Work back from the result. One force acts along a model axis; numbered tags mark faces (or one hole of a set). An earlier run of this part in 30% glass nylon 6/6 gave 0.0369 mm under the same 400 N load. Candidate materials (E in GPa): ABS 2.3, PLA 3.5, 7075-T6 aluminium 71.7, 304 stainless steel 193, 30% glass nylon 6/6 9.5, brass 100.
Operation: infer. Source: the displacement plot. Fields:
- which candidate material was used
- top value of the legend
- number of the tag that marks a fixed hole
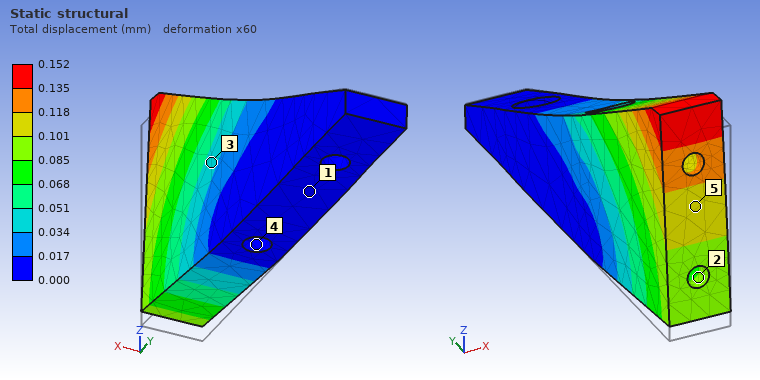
ABS
0.152 mm
4
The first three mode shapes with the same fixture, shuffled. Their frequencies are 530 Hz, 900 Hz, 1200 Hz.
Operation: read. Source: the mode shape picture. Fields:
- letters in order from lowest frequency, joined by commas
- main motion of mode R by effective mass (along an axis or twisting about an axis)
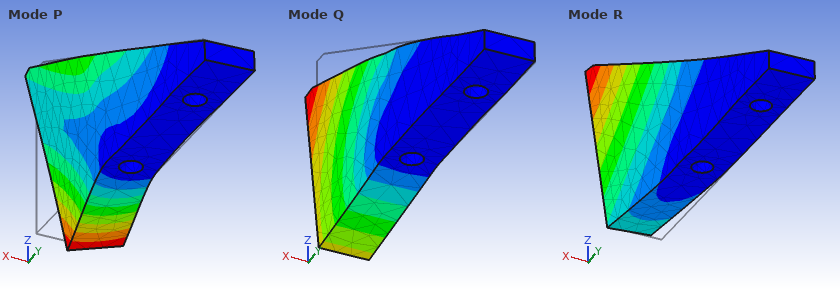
R, Q, P
along X
